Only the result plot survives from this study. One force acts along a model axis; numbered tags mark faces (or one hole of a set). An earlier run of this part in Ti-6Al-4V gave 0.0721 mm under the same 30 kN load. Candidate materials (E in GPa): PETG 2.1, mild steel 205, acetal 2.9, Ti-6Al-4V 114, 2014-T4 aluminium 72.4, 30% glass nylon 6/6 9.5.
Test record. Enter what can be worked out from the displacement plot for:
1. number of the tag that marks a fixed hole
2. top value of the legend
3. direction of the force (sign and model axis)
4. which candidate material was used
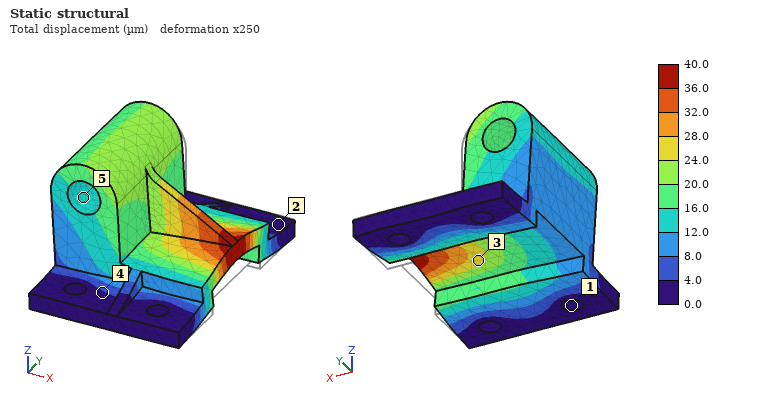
1
40.0 µm
+Z
mild steel
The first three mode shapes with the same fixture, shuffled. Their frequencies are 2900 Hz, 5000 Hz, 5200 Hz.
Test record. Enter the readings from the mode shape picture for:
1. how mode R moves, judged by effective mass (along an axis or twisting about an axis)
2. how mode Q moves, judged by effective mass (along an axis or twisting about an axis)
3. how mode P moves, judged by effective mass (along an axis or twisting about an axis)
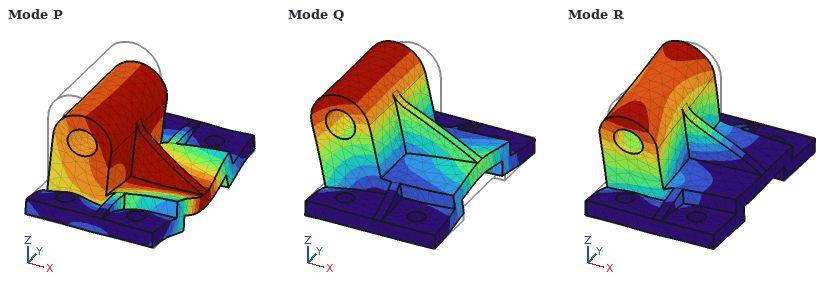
along Y
along X
along Z
